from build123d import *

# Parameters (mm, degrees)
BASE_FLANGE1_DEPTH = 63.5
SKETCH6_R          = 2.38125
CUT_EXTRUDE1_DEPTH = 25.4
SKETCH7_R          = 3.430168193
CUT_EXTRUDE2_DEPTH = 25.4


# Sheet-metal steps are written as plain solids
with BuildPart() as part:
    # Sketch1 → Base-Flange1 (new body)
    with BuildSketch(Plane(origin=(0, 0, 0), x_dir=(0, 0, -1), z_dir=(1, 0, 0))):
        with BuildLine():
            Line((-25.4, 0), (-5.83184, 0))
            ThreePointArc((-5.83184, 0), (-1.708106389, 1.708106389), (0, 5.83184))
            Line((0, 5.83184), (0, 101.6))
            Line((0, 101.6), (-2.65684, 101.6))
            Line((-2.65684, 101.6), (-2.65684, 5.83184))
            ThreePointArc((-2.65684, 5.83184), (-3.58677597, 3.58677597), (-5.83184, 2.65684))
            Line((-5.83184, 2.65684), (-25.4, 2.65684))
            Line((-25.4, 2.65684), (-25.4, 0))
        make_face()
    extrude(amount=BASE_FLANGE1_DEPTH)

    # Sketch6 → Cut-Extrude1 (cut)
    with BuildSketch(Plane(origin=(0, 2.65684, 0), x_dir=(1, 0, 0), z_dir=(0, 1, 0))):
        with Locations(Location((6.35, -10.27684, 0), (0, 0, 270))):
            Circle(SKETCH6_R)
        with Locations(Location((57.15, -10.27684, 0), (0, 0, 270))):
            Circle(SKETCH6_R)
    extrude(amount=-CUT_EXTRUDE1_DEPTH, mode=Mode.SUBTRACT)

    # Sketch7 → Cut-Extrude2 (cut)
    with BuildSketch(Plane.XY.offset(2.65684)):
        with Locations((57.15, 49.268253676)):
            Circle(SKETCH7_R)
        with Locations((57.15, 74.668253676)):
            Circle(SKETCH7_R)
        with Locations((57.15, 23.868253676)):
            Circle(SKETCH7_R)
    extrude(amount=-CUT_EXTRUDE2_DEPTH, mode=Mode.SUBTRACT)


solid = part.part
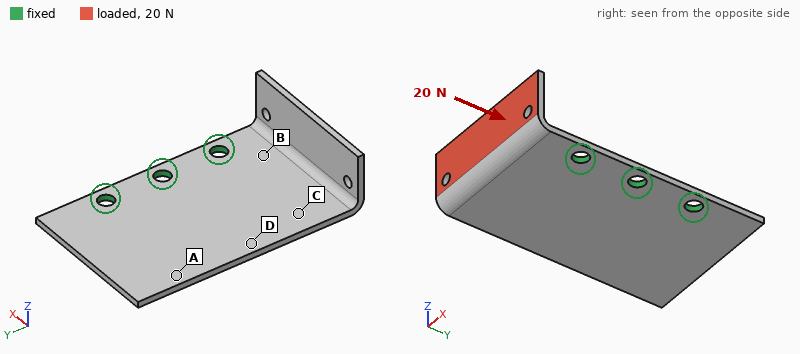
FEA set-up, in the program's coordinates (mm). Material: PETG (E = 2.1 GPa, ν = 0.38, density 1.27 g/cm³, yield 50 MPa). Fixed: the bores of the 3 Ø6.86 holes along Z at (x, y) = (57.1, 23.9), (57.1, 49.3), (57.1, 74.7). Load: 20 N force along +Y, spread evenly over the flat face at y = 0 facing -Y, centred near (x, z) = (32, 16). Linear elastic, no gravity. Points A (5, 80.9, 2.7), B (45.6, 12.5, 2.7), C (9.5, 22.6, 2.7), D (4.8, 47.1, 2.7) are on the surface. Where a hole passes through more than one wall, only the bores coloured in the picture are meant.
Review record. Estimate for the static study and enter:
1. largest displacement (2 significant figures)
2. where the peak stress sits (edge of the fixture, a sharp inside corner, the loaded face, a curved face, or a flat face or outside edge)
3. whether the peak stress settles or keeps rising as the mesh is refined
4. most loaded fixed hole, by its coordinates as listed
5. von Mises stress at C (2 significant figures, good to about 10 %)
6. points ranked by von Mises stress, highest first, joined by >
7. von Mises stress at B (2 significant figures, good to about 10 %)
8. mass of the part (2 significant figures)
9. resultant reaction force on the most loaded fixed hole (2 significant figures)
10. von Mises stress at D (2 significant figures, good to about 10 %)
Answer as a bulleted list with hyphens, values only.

- 1.4 mm
- edge of the fixture
- keeps rising
- (57.1, 23.9)
- 2.6 MPa
- B > C > D > A
- 4.1 MPa
- 26 g
- 14 N
- 1.2 MPa
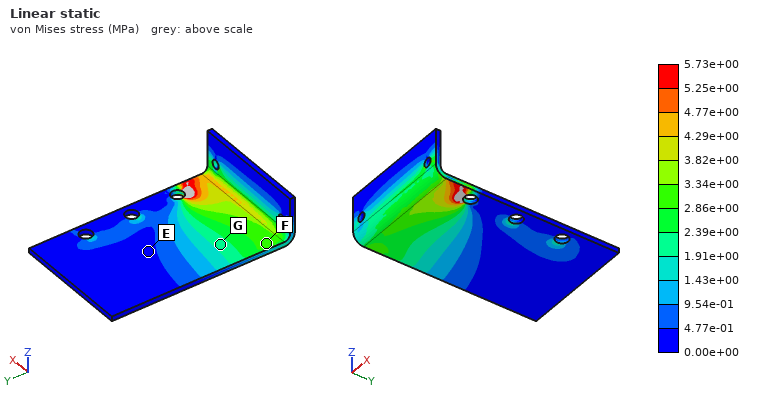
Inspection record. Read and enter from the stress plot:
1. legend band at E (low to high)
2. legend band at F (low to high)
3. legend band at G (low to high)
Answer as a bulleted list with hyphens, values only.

- 0.00e+00 to 4.77e-01 MPa
- 2.86e+00 to 3.34e+00 MPa
- 1.91e+00 to 2.39e+00 MPa
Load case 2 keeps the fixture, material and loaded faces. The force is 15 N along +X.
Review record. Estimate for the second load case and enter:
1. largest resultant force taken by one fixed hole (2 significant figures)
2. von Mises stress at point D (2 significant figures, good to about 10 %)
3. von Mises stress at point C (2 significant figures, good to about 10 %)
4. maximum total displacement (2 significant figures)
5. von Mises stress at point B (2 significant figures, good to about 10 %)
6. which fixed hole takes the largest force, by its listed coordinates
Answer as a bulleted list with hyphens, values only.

- 20 N
- 0.79 MPa
- 0.79 MPa
- 1.1 mm
- 2.1 MPa
- (57.1, 23.9)
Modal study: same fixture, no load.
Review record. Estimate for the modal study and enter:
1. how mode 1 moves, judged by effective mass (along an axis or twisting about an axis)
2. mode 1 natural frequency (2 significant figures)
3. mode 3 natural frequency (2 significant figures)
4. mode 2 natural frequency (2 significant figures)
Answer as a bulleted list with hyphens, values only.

- along Z
- 160 Hz
- 360 Hz
- 210 Hz
